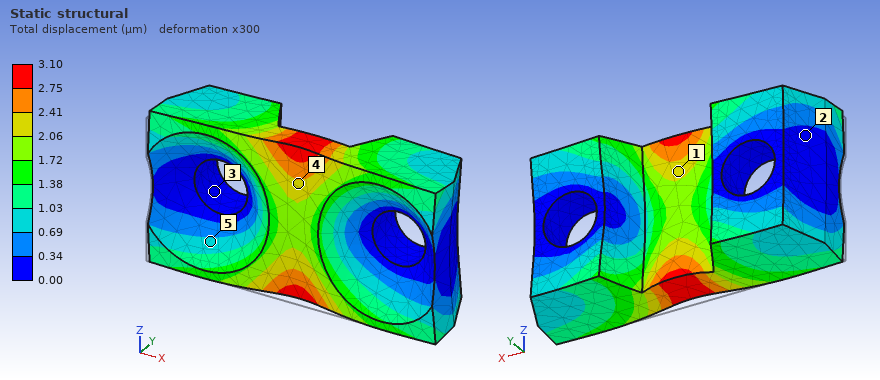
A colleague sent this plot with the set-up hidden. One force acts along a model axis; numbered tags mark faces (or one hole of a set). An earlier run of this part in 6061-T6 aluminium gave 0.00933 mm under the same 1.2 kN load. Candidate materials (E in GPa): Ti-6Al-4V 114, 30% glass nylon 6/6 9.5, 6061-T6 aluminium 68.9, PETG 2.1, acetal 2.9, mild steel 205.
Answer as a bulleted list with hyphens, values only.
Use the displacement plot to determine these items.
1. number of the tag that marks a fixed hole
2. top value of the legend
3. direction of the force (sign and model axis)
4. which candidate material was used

- 3
- 3.10 µm
- +Y
- mild steel
